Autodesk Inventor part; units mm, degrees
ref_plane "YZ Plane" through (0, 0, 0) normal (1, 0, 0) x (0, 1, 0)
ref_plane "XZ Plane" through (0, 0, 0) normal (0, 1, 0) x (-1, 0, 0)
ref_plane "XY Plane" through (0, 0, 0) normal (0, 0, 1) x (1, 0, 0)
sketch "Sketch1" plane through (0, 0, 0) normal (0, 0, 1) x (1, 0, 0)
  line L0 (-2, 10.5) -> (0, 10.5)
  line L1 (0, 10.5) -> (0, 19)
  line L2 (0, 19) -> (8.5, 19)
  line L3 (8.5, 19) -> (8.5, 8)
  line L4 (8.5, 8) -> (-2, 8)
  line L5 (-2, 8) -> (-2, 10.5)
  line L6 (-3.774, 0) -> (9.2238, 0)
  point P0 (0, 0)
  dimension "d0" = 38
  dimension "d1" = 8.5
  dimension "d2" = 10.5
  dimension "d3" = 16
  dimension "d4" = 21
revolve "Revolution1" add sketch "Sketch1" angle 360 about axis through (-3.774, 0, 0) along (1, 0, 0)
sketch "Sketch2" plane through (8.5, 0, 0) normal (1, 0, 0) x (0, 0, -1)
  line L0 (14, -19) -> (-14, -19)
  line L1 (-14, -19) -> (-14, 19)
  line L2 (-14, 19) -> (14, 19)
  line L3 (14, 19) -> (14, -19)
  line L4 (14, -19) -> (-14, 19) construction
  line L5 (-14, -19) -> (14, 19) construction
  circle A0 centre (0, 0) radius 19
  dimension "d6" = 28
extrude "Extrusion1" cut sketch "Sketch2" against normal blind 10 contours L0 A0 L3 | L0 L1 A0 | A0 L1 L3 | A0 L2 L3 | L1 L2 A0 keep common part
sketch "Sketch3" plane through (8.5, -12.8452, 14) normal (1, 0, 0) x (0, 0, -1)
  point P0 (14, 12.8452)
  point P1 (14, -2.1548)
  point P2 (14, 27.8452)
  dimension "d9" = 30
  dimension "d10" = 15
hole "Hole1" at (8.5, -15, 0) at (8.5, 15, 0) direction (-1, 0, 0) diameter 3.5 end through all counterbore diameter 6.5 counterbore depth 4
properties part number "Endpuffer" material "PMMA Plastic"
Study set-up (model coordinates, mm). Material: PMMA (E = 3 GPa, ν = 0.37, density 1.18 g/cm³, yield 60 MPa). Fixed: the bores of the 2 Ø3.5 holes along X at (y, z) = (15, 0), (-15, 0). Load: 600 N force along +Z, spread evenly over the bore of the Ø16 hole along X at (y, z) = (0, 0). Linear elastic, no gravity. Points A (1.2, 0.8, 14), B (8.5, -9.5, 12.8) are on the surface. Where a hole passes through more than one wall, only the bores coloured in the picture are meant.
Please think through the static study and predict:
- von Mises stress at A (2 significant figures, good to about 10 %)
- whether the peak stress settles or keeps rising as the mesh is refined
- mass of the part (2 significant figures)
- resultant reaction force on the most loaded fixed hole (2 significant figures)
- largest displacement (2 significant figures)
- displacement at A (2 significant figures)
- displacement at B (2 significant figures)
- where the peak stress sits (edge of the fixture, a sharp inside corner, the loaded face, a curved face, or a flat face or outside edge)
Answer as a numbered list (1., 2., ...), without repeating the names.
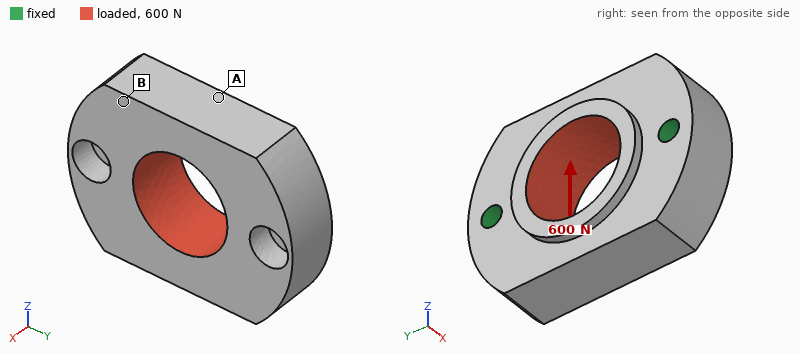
1. 4.9 MPa
2. keeps rising
3. 7.4 g
4. 300 N
5. 56 µm
6. 41 µm
7. 45 µm
8. edge of the fixture
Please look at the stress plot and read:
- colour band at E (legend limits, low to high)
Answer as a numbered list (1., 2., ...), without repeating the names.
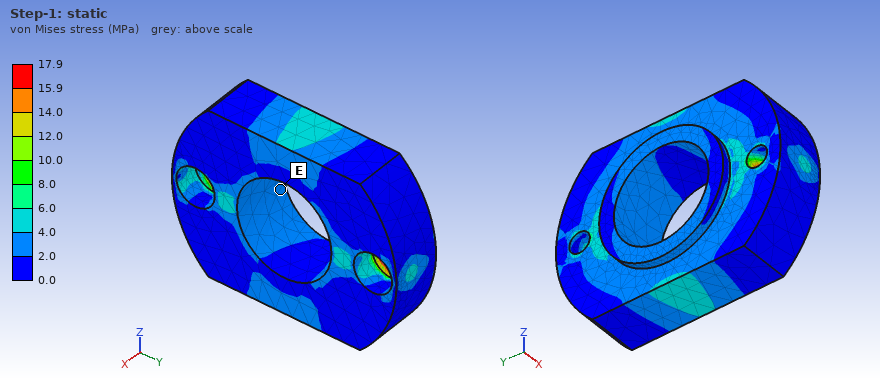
1. 2.0 to 4.0 MPa
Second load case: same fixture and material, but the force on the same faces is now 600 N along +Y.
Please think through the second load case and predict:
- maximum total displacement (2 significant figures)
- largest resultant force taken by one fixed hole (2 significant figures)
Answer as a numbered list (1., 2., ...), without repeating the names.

1. 25 µm
2. 300 N
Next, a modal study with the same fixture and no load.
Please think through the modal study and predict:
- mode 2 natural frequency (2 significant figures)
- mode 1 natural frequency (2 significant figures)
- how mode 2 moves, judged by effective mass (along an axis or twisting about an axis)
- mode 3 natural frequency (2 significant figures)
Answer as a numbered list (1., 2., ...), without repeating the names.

1. 5700 Hz
2. 3500 Hz
3. along X
4. 8200 Hz
